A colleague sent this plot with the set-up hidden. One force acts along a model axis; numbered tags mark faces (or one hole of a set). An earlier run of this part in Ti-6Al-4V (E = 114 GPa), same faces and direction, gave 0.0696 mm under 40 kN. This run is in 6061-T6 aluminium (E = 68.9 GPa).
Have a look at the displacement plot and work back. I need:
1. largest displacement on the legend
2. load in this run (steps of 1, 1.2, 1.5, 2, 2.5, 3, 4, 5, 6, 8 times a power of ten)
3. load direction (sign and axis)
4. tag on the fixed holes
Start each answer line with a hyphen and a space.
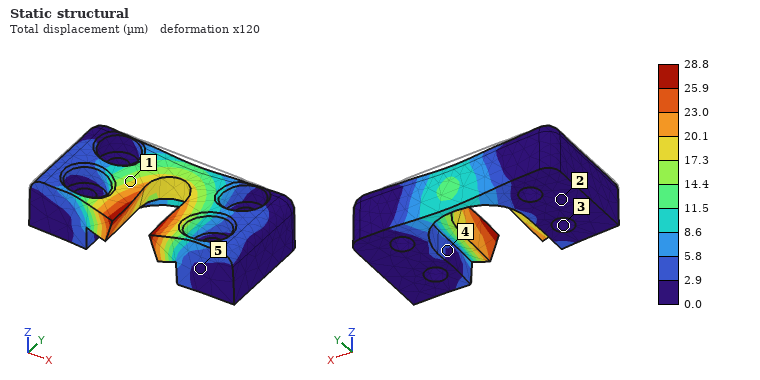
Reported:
- 28.8 µm
- 10 kN
- -Z
- 3
